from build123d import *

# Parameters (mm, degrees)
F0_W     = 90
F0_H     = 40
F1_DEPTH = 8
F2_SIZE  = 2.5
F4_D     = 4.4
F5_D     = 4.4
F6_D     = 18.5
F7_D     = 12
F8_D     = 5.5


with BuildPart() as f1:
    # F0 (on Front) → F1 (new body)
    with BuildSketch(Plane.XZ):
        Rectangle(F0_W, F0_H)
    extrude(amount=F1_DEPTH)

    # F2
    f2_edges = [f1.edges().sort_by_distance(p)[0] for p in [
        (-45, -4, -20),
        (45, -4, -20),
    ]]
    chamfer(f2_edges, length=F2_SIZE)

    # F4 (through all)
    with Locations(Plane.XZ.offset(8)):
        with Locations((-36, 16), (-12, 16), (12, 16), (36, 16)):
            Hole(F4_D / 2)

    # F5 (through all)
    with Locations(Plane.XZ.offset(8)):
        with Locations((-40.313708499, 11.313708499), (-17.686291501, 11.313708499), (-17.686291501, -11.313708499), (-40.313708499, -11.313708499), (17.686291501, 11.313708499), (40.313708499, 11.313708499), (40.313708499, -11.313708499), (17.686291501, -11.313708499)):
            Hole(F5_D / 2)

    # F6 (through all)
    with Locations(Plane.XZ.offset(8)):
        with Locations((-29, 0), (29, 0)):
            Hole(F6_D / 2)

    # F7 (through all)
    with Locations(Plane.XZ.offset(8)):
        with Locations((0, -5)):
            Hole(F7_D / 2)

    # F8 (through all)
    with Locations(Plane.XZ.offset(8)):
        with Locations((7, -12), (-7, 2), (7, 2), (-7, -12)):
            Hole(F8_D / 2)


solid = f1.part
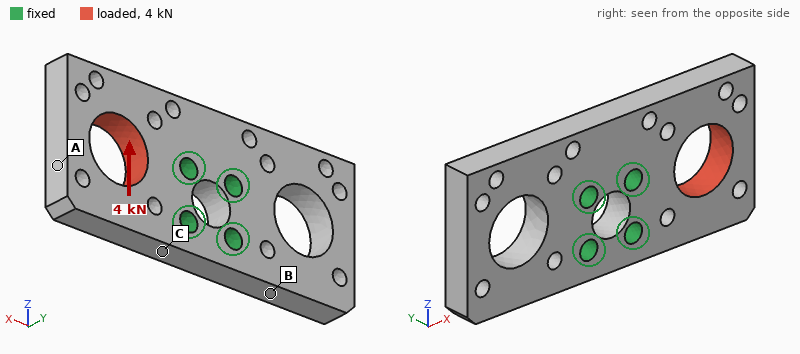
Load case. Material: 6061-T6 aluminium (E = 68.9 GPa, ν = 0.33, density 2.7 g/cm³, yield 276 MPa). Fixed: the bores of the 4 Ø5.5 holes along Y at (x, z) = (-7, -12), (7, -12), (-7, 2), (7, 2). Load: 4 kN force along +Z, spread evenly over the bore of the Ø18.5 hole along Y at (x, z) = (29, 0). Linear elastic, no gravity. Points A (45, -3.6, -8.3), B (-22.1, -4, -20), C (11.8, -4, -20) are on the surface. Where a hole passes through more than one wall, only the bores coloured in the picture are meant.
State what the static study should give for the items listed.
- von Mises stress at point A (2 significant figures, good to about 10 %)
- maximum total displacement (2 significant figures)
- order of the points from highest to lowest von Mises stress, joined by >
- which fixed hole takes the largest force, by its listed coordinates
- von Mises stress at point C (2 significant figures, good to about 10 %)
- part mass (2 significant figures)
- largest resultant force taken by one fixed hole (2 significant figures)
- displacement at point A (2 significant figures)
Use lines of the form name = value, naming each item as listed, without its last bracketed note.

von Mises stress at point A = 35 MPa
maximum total displacement = 63 µm
order of the points from highest to lowest von Mises stress, joined by > = C > A > B
which fixed hole takes the largest force, by its listed coordinates = (7, 2)
von Mises stress at point C = 54 MPa
part mass = 58 g
largest resultant force taken by one fixed hole = 4.1 kN
displacement at point A = 58 µm
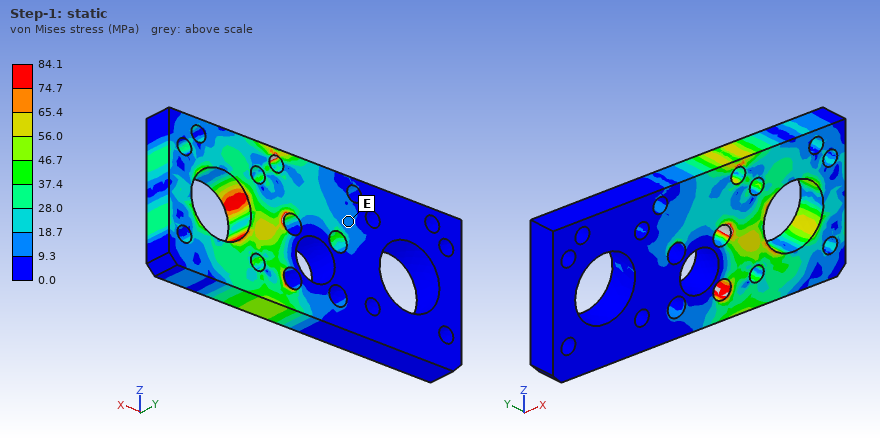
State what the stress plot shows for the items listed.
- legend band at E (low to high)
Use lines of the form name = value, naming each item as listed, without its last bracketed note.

legend band at E = 9.3 to 18.7 MPa
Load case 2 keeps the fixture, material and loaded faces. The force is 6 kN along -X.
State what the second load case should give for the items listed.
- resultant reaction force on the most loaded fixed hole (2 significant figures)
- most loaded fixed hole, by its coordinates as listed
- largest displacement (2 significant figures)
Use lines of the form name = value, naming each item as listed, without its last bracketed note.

resultant reaction force on the most loaded fixed hole = 3.1 kN
most loaded fixed hole, by its coordinates as listed = (7, 2)
largest displacement = 28 µm
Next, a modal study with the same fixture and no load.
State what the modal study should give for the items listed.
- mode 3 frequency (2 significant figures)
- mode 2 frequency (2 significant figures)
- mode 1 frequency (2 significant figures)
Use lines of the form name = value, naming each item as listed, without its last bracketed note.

mode 3 frequency = 7500 Hz
mode 2 frequency = 4200 Hz
mode 1 frequency = 4200 Hz
